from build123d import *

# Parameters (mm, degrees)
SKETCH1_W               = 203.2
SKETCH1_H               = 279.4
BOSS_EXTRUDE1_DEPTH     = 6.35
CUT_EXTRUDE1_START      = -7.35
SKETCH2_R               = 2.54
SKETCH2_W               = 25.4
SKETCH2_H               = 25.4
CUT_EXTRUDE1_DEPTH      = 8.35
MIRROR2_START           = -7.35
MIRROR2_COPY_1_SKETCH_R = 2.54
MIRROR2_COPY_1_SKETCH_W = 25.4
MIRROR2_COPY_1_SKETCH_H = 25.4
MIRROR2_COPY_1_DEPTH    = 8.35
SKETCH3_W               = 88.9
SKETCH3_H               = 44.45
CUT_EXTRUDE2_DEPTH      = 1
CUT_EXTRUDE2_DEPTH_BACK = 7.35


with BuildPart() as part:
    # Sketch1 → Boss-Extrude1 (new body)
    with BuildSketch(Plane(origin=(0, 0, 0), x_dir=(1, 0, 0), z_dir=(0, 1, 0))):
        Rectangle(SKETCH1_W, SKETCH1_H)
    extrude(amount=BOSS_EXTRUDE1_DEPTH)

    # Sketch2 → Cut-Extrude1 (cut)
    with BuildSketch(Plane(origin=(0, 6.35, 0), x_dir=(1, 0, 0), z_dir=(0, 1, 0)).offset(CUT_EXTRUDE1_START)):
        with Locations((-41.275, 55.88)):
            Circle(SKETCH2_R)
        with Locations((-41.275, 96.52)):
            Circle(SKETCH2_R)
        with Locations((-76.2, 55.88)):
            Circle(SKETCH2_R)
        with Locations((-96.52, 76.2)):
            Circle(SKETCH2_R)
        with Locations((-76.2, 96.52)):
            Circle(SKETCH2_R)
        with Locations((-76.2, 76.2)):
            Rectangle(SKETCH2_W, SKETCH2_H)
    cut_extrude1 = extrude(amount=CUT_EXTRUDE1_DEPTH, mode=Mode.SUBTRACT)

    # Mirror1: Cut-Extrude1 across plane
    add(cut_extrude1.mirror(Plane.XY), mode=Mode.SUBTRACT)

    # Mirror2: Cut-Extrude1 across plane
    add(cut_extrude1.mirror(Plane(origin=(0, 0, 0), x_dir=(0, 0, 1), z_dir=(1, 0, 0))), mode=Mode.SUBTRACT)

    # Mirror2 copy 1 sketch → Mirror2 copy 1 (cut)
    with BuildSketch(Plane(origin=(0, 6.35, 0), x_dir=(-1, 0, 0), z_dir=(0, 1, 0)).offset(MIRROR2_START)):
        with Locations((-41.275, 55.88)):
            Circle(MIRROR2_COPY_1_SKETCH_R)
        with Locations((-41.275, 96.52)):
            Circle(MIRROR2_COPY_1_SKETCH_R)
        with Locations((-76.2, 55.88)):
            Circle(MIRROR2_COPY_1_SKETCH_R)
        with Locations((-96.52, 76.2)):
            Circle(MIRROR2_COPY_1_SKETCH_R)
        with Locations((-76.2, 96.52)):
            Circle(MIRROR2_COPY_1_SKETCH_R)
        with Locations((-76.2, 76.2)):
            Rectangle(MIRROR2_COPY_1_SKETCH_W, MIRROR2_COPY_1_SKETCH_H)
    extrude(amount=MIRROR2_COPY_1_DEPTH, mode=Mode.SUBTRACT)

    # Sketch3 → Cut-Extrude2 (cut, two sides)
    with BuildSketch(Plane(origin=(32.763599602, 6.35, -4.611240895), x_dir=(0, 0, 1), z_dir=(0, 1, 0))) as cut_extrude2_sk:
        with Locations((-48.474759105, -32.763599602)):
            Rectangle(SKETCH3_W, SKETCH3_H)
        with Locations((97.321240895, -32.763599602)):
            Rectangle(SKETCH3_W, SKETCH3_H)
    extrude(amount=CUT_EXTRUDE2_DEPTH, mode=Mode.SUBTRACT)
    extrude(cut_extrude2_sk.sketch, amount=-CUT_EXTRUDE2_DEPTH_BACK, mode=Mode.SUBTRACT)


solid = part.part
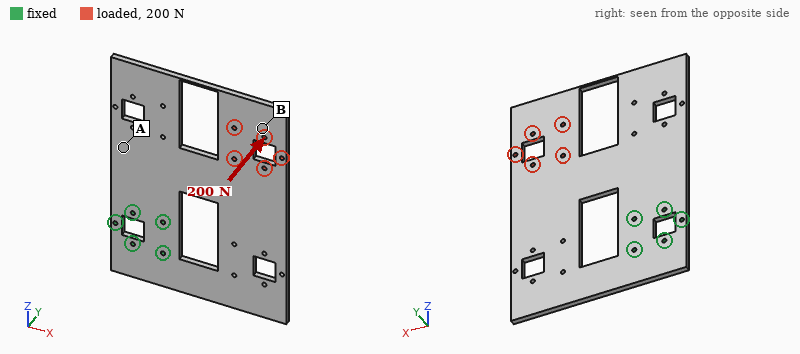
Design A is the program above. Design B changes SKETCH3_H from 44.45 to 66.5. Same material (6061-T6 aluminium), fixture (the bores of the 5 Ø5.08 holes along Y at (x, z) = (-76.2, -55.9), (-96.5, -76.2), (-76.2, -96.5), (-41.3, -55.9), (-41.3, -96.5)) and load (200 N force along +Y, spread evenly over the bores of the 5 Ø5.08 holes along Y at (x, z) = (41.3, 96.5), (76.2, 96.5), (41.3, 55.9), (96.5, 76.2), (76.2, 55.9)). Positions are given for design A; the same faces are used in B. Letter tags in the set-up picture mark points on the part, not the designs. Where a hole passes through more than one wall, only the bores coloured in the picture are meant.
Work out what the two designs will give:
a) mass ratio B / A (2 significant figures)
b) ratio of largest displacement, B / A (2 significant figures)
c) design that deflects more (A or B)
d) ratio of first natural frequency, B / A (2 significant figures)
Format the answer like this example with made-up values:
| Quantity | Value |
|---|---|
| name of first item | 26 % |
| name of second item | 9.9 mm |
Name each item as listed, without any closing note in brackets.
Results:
| Quantity | Value |
|---|---|
| mass ratio B / A | 0.91 |
| ratio of largest displacement, B / A | 1.2 |
| design that deflects more | B |
| ratio of first natural frequency, B / A | 0.94 |
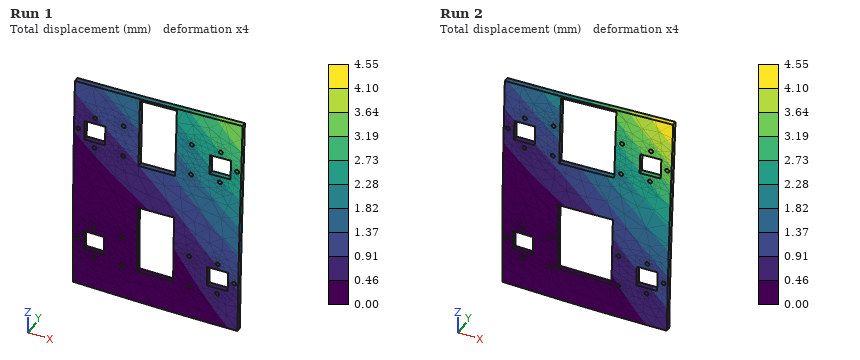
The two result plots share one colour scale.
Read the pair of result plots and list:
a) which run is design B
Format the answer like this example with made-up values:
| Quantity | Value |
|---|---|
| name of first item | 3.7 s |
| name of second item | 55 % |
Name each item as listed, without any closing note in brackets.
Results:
| Quantity | Value |
|---|---|
| which run is design B | Run 2 |
